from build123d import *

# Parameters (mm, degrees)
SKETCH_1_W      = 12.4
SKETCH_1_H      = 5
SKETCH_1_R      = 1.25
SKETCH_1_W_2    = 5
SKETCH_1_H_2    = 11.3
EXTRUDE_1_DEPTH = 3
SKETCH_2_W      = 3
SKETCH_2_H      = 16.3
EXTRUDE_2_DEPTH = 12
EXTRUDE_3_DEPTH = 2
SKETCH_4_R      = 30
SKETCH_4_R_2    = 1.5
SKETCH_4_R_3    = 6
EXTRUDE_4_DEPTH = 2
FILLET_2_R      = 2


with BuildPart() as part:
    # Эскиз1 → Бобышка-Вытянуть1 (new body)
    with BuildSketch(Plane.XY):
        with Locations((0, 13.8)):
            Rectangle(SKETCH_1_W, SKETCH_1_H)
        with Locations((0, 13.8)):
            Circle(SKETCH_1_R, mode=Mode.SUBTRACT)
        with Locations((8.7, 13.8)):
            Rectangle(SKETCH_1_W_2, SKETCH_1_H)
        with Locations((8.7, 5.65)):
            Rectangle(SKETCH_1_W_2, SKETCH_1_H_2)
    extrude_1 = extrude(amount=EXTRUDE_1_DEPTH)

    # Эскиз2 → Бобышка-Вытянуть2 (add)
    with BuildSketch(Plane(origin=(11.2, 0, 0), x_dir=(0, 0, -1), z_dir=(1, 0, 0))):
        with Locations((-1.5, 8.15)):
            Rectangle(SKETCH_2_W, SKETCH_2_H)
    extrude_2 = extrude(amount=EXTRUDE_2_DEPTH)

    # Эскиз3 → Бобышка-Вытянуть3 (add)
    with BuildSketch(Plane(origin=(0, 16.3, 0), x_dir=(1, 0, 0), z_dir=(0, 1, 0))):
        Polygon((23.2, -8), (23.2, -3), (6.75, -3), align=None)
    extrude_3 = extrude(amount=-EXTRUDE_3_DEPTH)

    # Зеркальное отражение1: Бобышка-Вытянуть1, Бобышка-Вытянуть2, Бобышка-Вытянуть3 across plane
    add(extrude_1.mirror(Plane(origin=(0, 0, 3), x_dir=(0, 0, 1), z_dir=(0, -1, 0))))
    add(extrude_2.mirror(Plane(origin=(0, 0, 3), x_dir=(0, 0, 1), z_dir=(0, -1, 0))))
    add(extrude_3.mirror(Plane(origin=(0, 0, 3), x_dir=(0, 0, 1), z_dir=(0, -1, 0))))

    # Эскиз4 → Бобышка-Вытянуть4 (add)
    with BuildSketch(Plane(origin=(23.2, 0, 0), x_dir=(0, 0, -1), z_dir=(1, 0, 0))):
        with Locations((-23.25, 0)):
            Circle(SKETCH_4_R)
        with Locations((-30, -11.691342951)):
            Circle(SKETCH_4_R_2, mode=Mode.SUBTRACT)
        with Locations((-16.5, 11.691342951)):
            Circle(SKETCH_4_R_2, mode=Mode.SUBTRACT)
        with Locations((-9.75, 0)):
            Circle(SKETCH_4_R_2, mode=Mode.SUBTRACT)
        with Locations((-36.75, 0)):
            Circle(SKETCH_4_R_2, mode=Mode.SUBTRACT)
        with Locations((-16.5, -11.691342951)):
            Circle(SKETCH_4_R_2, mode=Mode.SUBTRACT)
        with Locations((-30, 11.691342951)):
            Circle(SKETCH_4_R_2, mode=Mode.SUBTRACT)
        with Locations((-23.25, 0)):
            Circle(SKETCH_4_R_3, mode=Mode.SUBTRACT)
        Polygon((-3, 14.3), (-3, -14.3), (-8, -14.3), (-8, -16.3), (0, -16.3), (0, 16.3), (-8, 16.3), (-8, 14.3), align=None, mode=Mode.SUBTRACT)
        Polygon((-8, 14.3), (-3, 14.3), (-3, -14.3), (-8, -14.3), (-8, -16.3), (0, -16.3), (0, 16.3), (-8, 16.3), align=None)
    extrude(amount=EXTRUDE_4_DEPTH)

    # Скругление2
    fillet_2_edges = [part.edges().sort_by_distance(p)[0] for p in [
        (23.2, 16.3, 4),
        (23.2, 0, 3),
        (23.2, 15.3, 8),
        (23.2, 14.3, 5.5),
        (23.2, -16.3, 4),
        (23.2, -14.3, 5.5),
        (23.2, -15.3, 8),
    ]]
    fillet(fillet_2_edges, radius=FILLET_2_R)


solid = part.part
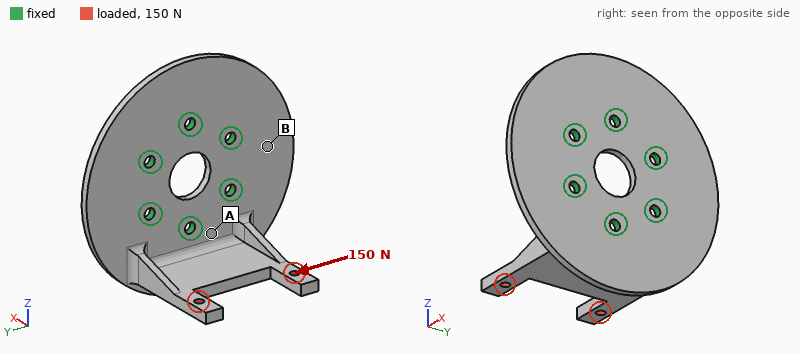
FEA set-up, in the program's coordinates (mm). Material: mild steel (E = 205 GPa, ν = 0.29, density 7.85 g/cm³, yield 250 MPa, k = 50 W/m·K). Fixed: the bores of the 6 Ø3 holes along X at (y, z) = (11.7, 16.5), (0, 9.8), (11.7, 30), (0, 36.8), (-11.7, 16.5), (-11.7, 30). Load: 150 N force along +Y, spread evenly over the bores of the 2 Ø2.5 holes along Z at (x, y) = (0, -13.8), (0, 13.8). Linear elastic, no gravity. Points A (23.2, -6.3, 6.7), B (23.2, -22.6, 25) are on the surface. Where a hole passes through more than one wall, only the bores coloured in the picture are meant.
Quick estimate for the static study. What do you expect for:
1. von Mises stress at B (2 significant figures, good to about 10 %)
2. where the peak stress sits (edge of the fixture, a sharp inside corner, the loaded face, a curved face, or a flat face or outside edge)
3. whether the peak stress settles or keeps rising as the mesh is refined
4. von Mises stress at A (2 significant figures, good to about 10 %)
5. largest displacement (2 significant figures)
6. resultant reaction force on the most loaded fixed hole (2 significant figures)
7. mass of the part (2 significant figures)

9.8 MPa
edge of the fixture
keeps rising
22 MPa
43 µm
130 N
59 g
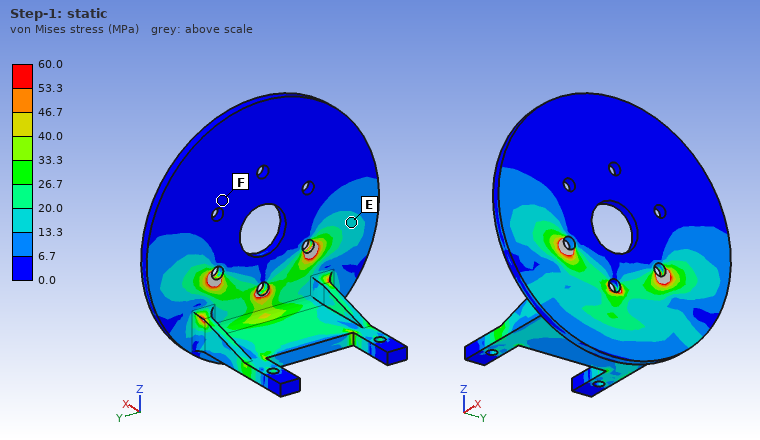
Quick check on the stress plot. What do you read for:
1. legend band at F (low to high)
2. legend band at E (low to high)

0.0 to 6.7 MPa
13.3 to 20.0 MPa
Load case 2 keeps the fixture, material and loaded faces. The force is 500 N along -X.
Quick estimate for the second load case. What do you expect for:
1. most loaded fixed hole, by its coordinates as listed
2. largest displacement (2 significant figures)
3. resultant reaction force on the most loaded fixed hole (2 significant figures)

(0, 9.8)
90 µm
590 N
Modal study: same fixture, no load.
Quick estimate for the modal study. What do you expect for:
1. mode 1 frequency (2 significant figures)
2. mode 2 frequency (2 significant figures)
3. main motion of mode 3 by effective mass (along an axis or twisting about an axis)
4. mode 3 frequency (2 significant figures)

2500 Hz
3600 Hz
along X
5800 Hz
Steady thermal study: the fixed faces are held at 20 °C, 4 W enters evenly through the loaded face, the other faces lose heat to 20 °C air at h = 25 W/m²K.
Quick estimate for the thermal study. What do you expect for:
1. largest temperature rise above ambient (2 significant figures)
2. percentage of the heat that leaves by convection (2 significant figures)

43 K
27 %
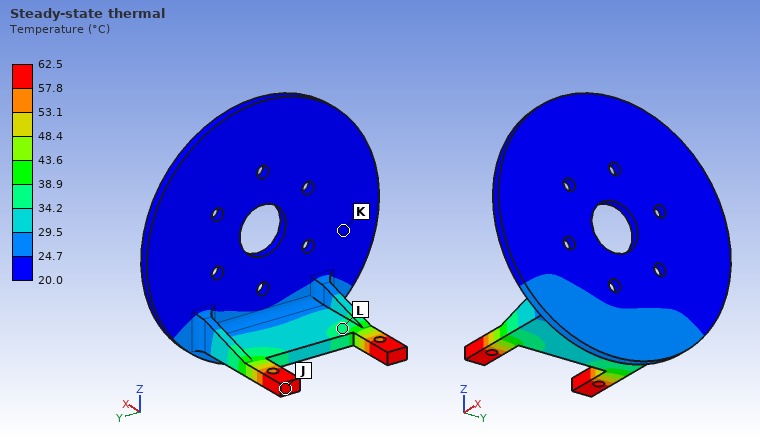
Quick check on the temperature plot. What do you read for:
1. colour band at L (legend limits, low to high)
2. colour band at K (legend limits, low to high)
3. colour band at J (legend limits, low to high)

34.2 to 38.9 °C
20.0 to 24.7 °C
57.8 to 62.5 °C
